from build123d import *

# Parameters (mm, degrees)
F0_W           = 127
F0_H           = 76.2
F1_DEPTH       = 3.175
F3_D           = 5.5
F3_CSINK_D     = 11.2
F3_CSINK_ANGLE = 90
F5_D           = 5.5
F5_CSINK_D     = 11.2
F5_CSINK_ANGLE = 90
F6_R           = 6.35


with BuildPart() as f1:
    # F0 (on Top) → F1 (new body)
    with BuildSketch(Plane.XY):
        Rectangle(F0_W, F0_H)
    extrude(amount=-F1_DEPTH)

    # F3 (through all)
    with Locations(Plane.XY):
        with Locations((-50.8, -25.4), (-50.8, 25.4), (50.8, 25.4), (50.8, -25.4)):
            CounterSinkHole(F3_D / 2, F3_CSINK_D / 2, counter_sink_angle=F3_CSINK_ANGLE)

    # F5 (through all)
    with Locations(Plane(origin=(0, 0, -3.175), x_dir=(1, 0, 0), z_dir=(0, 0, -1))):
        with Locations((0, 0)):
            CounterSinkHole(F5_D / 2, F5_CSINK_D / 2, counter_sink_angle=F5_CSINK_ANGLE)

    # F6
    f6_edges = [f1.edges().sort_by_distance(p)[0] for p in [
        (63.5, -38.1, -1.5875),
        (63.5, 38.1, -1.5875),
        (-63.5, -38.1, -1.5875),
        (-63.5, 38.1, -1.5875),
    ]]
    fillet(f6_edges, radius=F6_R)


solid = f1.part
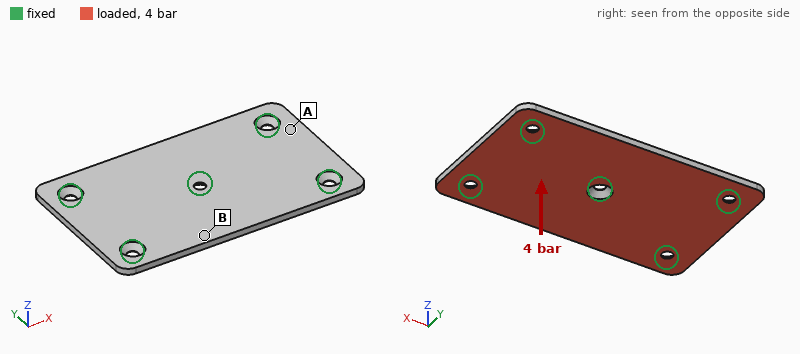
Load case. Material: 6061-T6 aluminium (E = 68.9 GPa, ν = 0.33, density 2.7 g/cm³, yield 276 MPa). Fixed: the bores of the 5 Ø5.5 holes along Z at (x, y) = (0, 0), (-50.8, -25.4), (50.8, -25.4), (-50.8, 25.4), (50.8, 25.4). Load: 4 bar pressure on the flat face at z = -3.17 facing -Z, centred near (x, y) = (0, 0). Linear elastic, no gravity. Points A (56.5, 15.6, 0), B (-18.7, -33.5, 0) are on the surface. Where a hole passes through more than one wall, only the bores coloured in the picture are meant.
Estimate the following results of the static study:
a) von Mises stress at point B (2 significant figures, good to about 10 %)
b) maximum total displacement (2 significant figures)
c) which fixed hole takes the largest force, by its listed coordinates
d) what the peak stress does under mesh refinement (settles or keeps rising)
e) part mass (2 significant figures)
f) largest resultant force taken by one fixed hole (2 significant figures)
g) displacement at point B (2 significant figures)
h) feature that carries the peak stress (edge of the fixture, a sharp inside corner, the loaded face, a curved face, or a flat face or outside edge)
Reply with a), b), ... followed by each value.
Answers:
a) 51 MPa
b) 0.34 mm
c) (0, 0)
d) keeps rising
e) 80 g
f) 1.4 kN
g) 0.25 mm
h) edge of the fixture
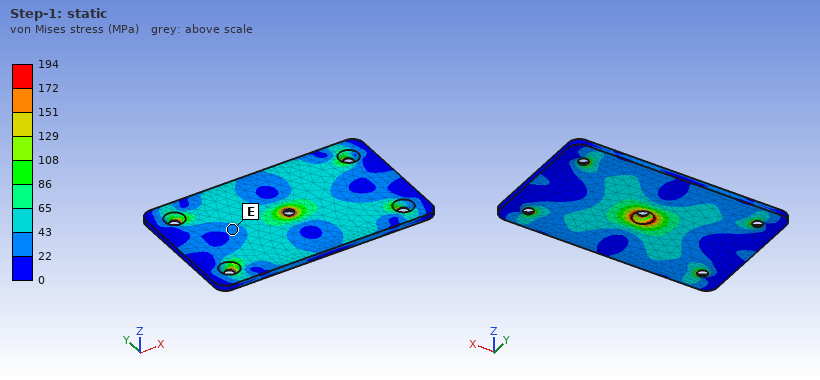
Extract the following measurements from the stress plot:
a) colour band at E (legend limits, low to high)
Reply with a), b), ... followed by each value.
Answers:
a) 22 to 43 MPa
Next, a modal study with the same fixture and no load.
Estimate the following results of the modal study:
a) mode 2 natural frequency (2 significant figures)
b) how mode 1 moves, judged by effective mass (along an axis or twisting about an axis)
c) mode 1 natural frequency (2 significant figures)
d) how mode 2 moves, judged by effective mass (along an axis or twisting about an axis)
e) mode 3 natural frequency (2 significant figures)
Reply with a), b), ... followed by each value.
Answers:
a) 2400 Hz
b) twisting about X
c) 2000 Hz
d) along Z
e) 3300 Hz
